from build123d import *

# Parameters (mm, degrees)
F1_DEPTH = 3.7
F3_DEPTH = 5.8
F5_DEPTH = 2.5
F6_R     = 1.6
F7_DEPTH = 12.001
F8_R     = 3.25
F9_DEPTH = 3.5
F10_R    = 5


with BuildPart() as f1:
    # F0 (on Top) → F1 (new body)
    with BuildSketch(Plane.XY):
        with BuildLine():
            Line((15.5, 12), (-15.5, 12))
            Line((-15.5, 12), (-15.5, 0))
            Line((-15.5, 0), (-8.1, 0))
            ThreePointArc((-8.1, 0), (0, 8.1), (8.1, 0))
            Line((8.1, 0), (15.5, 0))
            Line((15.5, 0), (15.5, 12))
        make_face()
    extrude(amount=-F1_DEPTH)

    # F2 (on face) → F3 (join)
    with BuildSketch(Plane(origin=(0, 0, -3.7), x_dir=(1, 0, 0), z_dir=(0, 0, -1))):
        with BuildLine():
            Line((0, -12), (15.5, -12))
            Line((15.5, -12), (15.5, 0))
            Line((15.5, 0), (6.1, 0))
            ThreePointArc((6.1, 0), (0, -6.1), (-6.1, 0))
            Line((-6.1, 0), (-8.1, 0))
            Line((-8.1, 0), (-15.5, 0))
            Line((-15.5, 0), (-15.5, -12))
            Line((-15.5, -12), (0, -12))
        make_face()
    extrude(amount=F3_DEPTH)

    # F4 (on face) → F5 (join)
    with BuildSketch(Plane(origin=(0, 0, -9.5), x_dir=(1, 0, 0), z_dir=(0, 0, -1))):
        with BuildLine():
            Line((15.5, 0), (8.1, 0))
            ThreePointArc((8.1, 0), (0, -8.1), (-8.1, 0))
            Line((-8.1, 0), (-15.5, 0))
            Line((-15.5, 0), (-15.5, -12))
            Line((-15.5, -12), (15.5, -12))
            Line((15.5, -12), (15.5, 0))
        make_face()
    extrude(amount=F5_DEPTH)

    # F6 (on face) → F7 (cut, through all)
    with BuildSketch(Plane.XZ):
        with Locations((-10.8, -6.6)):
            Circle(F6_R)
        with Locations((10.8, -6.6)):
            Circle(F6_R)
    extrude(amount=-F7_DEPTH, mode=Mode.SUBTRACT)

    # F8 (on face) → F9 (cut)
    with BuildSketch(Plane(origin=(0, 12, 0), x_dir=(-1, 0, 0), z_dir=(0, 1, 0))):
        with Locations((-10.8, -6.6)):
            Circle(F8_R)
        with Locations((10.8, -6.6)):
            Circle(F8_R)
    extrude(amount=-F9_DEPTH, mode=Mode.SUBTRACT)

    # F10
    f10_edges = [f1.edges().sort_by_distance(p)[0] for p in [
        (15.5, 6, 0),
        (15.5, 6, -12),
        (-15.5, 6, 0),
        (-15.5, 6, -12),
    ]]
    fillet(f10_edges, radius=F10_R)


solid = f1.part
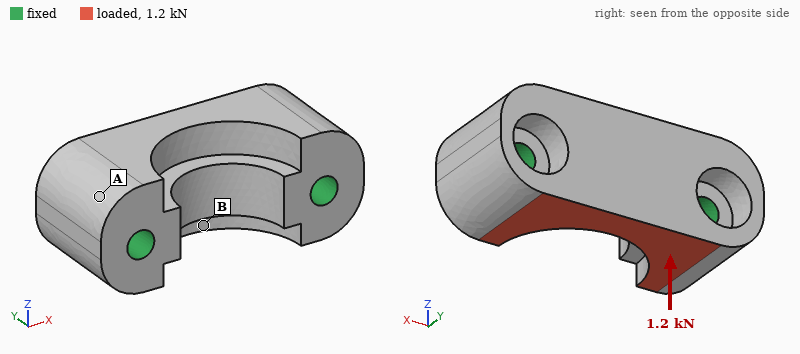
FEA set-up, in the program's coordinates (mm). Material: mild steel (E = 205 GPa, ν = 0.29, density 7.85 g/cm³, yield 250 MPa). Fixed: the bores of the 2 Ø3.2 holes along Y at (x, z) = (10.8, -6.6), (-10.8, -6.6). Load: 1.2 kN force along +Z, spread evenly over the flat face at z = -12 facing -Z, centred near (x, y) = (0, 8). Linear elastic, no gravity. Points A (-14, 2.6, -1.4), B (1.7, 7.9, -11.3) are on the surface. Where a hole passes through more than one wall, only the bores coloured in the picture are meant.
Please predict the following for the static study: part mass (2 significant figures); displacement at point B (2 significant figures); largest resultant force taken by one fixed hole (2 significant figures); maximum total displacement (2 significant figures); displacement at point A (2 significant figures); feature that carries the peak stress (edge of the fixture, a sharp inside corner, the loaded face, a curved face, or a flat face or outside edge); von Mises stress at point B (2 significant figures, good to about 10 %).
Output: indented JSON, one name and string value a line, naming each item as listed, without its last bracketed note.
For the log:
{
  "part mass": "22 g",
  "displacement at point B": "1.3 µm",
  "largest resultant force taken by one fixed hole": "600 N",
  "maximum total displacement": "1.9 µm",
  "displacement at point A": "0.34 µm",
  "feature that carries the peak stress": "edge of the fixture",
  "von Mises stress at point B": "13 MPa"
}
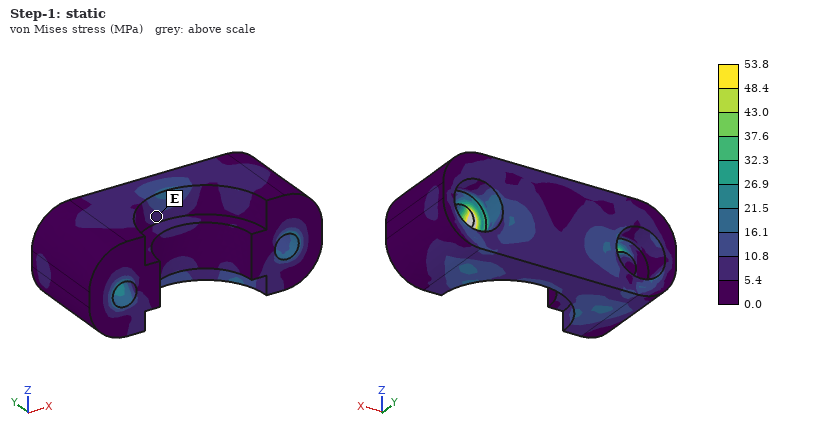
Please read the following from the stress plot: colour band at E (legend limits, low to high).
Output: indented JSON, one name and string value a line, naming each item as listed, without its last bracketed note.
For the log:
{
  "colour band at E": "5.4 to 10.8 MPa"
}
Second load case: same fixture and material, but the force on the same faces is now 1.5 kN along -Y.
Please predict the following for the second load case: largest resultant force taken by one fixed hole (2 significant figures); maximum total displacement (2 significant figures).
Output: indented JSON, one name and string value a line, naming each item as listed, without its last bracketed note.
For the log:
{
  "largest resultant force taken by one fixed hole": "800 N",
  "maximum total displacement": "3.7 µm"
}
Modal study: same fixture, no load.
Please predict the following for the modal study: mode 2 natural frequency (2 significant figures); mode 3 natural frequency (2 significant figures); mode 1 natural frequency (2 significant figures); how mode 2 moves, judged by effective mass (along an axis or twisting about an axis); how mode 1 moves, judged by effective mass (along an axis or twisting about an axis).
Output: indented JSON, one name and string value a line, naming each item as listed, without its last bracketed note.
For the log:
{
  "mode 2 natural frequency": "61 kHz",
  "mode 3 natural frequency": "69 kHz",
  "mode 1 natural frequency": "41 kHz",
  "how mode 2 moves, judged by effective mass": "along Y",
  "how mode 1 moves, judged by effective mass": "along Z"
}
